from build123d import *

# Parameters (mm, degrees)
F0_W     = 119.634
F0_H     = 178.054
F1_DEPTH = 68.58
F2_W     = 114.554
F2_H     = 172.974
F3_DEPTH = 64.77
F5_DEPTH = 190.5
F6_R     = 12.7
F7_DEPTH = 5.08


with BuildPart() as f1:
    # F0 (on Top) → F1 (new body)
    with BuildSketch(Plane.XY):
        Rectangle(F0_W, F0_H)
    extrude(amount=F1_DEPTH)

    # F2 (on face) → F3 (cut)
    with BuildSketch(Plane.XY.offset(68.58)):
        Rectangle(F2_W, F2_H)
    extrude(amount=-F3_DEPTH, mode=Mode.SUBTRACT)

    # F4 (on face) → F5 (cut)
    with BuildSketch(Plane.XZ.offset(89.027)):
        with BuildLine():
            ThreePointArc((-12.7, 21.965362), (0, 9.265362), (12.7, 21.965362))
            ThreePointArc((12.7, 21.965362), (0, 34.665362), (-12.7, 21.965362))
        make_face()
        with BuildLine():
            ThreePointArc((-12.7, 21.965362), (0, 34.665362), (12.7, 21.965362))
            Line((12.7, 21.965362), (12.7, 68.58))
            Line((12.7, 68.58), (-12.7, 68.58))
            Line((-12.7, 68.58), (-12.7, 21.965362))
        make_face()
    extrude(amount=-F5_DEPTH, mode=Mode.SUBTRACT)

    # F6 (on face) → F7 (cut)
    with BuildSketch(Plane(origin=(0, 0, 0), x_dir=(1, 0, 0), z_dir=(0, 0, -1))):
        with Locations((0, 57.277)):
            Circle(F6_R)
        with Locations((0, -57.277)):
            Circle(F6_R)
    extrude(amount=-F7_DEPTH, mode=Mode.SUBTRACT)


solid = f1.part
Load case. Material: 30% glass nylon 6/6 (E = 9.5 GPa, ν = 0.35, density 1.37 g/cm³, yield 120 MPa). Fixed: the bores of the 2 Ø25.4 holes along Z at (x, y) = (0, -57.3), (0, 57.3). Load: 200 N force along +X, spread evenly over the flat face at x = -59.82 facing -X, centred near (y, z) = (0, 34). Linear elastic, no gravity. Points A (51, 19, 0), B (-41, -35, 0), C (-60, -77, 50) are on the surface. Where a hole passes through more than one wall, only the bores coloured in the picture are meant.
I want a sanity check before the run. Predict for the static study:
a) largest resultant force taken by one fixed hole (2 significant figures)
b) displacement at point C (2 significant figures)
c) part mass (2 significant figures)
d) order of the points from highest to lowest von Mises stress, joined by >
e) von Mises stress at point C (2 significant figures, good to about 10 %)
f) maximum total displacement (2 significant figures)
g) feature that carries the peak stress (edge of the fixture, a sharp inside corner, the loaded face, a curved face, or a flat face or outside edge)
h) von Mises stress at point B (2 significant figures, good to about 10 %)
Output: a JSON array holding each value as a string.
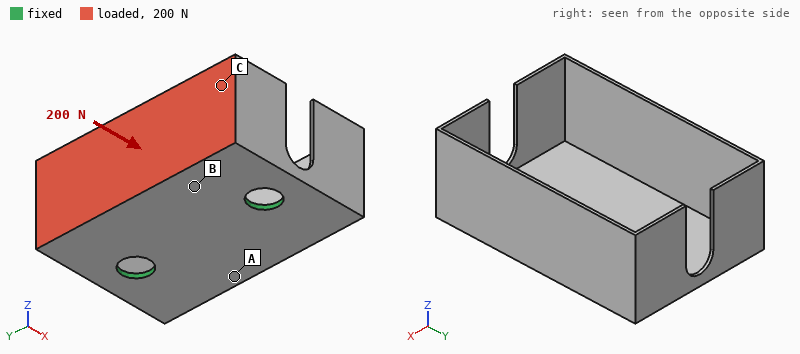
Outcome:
["130 N", "0.74 mm", "230 g", "C > B > A", "8.2 MPa", "2.5 mm", "a curved face", "5.5 MPa"]
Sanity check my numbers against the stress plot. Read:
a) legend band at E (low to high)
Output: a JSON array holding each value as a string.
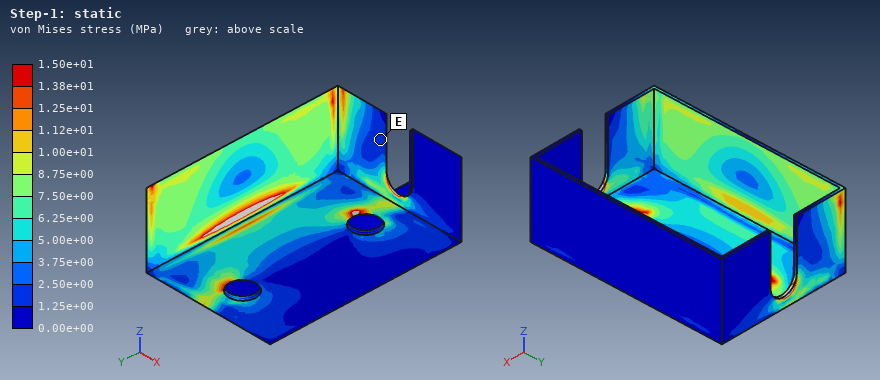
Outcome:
["1.25e+00 to 2.50e+00 MPa"]
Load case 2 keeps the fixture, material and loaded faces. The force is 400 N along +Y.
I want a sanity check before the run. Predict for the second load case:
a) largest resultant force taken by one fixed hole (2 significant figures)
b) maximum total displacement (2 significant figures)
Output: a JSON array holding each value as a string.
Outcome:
["280 N", "1.2 mm"]
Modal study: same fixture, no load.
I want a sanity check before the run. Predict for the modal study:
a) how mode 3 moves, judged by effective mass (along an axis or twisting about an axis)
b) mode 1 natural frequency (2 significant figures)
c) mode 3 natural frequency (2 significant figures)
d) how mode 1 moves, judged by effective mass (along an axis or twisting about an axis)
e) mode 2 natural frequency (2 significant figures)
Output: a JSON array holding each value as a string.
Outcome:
["along Z", "240 Hz", "280 Hz", "along X", "260 Hz"]
